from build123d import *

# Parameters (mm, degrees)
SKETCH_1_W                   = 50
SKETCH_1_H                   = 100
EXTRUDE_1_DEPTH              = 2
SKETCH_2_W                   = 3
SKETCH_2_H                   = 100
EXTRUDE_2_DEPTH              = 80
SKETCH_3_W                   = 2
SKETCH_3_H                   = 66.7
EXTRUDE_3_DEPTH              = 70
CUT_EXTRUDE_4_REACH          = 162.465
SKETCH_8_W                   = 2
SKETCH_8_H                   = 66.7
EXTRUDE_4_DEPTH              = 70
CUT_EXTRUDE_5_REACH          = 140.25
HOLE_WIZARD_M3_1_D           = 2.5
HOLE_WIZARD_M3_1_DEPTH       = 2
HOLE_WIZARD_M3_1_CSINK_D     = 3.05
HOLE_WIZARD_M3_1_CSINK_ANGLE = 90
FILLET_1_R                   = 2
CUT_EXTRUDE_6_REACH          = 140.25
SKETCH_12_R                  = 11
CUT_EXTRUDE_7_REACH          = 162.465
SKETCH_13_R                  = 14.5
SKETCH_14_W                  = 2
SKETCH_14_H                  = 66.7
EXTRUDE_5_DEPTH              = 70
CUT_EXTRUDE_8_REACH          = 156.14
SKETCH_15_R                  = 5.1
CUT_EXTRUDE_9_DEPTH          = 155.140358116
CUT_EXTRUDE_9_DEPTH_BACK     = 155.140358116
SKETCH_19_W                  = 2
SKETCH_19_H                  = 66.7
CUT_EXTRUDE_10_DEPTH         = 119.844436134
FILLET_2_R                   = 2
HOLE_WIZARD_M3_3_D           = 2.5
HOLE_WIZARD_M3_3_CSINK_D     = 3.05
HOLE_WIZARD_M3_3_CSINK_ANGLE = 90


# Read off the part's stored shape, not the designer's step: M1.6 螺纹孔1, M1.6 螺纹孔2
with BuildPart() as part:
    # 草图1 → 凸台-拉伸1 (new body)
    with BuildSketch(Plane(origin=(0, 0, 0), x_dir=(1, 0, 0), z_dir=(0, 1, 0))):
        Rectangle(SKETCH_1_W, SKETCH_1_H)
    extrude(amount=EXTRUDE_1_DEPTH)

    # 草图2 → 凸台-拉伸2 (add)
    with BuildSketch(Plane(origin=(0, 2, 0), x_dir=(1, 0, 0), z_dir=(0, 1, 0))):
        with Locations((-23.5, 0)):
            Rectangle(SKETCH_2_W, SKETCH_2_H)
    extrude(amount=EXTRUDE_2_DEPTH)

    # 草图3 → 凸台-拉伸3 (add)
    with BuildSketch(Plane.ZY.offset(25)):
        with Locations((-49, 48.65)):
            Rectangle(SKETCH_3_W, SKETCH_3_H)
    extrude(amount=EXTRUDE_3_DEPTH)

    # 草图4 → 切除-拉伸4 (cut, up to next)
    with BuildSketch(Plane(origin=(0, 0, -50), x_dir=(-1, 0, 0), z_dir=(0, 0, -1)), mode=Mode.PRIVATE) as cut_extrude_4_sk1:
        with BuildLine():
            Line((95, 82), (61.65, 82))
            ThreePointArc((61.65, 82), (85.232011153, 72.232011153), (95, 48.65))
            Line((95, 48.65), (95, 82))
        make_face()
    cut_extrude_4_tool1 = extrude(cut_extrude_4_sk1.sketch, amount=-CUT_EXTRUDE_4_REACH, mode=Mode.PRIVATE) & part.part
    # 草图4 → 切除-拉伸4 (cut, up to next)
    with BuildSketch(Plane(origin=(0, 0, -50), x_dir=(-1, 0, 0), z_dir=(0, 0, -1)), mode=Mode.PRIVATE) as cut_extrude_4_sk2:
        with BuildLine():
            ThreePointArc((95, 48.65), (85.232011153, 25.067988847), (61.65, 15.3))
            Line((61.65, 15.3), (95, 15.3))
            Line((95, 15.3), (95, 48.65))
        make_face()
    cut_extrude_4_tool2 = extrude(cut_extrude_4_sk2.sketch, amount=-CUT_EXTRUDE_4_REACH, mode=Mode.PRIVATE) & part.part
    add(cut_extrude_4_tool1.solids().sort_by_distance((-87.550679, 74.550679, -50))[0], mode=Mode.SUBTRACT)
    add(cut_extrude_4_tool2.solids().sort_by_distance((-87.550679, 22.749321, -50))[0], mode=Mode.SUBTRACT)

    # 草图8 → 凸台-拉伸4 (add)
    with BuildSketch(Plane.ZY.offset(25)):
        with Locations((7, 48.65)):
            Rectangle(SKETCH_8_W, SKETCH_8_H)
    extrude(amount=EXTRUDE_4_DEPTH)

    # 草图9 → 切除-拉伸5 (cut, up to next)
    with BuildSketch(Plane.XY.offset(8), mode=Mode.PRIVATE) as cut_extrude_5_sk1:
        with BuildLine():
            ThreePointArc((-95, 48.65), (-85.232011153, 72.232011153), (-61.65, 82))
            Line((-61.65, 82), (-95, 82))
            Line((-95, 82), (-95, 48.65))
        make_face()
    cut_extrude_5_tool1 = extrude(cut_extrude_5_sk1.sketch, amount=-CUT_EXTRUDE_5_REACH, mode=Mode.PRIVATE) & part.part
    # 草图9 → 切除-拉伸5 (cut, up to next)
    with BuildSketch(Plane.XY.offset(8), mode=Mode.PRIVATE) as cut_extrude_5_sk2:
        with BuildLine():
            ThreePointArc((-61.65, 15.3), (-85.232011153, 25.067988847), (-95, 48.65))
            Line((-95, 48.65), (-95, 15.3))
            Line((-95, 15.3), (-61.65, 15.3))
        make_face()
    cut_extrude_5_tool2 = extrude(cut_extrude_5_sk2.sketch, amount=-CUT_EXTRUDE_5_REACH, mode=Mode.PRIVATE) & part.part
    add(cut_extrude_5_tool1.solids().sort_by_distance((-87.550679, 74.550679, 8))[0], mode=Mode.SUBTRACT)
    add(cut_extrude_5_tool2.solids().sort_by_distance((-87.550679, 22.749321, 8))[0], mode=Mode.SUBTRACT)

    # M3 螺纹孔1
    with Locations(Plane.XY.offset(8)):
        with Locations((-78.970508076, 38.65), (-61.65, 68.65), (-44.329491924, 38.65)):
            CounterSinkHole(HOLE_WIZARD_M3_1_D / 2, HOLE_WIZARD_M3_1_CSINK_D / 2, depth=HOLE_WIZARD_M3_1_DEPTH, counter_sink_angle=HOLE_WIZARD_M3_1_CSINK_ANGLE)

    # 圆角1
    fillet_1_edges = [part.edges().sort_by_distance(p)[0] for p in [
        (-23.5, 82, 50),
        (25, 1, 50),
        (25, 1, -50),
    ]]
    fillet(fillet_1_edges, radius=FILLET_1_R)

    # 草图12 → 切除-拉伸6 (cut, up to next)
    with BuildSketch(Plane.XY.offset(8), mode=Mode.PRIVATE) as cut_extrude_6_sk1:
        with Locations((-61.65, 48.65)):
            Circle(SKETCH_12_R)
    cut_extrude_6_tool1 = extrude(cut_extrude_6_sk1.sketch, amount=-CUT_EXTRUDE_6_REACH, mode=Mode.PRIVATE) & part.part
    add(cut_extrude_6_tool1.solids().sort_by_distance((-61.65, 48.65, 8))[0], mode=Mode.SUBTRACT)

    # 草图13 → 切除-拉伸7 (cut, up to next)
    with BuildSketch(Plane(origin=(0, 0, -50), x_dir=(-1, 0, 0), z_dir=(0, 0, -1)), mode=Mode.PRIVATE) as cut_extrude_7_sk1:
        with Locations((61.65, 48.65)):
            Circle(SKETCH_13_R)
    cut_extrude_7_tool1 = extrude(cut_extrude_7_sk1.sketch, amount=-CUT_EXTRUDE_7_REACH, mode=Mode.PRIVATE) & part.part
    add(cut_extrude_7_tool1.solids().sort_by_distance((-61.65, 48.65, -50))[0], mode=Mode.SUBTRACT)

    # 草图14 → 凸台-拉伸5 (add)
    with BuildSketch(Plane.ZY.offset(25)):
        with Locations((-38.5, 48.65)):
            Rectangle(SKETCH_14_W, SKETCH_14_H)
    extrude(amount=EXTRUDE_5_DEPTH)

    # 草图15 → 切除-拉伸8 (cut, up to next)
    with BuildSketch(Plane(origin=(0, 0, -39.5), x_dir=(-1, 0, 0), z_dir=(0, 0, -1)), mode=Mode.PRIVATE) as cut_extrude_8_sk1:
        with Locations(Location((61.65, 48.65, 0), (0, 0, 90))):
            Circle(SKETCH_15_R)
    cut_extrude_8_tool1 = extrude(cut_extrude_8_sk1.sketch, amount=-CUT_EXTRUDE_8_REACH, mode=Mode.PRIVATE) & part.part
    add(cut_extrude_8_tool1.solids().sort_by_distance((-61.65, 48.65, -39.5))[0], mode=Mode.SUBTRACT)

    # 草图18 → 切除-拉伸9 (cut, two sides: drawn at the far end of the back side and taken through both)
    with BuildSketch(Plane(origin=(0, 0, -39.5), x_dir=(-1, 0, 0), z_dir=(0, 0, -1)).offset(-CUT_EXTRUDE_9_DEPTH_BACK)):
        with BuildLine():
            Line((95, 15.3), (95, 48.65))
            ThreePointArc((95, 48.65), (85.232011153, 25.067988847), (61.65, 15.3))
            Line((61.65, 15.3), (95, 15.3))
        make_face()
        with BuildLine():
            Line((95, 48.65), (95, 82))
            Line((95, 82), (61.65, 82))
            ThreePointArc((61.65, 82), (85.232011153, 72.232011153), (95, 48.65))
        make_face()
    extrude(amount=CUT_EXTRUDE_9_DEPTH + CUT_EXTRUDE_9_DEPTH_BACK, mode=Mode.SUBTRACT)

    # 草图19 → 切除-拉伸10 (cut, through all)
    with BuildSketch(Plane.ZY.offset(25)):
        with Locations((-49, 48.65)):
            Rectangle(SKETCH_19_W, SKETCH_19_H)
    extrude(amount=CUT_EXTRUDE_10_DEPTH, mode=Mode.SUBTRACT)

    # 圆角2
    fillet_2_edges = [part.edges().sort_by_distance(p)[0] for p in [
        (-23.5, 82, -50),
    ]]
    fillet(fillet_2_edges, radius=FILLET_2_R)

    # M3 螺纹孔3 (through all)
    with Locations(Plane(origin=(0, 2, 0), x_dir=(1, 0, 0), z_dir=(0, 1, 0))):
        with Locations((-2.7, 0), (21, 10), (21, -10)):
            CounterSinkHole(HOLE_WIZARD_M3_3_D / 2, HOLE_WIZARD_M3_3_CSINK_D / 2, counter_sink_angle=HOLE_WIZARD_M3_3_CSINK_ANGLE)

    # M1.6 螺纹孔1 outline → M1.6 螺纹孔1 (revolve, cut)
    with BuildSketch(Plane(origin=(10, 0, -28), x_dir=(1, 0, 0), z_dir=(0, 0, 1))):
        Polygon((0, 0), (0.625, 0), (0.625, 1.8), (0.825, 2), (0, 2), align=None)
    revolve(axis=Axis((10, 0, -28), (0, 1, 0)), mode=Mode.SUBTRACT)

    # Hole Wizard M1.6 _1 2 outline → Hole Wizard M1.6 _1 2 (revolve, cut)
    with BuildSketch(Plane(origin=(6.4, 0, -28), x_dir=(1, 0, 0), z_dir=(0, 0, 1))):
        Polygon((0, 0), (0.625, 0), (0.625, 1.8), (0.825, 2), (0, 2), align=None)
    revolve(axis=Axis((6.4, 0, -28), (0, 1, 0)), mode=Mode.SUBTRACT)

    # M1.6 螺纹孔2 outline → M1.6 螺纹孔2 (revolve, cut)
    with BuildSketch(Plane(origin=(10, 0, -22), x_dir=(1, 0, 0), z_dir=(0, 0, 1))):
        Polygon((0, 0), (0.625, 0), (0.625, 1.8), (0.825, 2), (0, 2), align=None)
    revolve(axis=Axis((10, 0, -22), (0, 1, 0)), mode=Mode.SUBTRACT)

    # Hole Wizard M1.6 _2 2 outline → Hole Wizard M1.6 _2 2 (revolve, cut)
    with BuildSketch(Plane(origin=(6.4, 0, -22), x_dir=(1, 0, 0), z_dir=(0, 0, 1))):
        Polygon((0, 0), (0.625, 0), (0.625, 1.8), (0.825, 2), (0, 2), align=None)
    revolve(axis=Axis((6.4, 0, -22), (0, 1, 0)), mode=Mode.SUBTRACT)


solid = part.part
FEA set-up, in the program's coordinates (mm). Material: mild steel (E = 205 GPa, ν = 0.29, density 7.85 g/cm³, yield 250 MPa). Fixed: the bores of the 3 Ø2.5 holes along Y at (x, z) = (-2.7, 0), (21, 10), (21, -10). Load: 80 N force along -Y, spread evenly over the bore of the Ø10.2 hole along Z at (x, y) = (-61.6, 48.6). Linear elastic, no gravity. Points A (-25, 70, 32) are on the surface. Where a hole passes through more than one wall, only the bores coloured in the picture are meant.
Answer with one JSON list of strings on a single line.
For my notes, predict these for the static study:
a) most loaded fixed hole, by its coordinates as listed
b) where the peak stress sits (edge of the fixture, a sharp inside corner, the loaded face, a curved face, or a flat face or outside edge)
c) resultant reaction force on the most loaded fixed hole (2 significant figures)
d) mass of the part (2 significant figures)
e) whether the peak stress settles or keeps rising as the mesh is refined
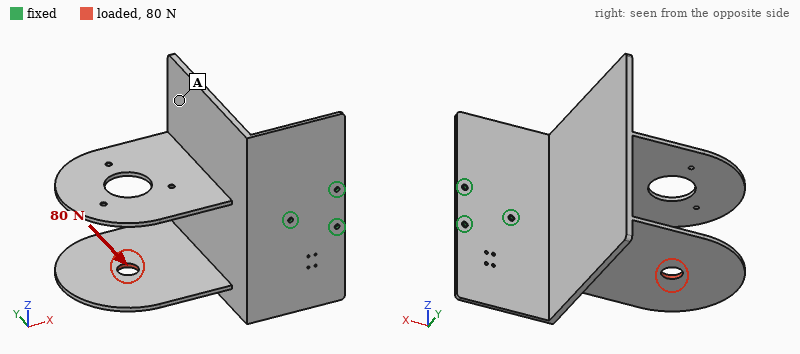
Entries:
["(-2.7, 0)", "edge of the fixture", "220 N", "390 g", "keeps rising"]
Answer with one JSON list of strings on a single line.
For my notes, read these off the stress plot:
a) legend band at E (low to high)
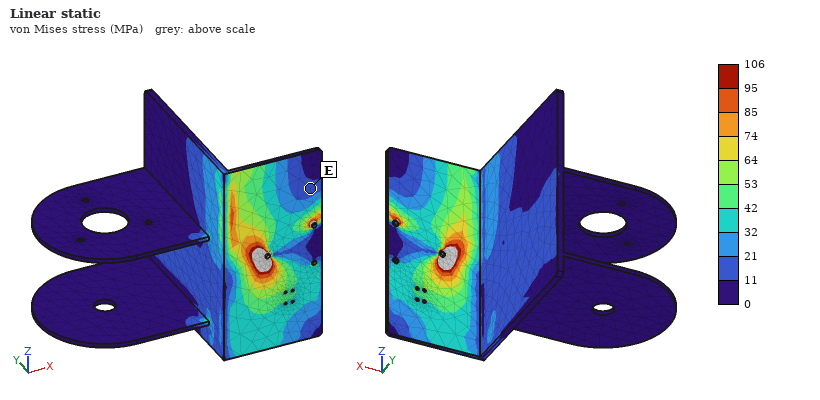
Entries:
["11 to 21 MPa"]
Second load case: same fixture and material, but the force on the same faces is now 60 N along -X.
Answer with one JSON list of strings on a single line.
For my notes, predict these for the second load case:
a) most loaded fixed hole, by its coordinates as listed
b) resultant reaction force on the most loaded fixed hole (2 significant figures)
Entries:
["(-2.7, 0)", "120 N"]
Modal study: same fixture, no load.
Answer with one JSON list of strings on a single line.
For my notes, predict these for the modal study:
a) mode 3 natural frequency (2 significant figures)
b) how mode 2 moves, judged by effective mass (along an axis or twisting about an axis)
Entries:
["320 Hz", "along Z"]
